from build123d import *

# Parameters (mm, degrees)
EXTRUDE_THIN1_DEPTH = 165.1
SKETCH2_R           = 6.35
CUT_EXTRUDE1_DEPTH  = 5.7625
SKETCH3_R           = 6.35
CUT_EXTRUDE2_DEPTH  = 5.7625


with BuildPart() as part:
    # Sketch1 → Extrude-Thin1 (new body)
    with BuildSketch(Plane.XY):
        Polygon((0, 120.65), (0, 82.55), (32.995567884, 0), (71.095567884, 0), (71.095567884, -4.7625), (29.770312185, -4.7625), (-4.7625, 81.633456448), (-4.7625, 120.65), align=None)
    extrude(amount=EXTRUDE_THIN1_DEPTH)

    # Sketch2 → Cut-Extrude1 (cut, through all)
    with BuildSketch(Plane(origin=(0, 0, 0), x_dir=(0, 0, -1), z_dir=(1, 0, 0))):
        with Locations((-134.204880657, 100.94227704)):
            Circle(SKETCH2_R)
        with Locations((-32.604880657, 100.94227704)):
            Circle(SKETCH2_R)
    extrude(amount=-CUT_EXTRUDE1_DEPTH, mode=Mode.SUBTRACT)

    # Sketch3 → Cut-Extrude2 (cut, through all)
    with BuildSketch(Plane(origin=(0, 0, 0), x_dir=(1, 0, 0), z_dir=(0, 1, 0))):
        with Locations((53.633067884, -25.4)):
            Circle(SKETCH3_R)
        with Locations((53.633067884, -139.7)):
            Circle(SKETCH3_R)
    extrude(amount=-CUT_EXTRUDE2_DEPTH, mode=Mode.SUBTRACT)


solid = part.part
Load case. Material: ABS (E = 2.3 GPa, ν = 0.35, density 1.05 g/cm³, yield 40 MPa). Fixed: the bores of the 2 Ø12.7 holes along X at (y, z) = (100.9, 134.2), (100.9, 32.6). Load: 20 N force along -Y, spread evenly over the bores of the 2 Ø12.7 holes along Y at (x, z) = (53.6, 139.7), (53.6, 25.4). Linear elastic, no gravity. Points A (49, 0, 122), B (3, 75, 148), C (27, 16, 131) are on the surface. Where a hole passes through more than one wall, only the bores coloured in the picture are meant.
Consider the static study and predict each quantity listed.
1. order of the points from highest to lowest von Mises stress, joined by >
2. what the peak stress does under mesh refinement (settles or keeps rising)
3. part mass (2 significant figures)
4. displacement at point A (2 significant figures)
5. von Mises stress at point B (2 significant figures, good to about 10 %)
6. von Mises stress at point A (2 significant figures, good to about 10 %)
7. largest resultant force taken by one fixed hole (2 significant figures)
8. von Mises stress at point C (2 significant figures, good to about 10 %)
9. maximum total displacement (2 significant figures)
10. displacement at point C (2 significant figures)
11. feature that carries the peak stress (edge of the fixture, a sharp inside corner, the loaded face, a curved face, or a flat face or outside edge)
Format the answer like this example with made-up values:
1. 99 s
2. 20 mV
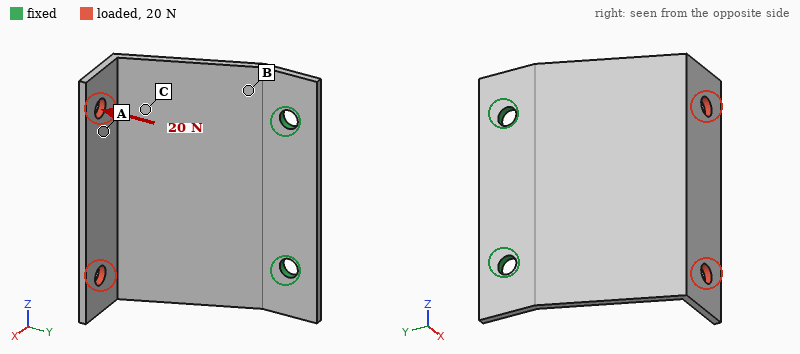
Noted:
1. B > C > A
2. keeps rising
3. 140 g
4. 1.8 mm
5. 1.7 MPa
6. 0.36 MPa
7. 11 N
8. 0.93 MPa
9. 2.3 mm
10. 1.2 mm
11. edge of the fixture
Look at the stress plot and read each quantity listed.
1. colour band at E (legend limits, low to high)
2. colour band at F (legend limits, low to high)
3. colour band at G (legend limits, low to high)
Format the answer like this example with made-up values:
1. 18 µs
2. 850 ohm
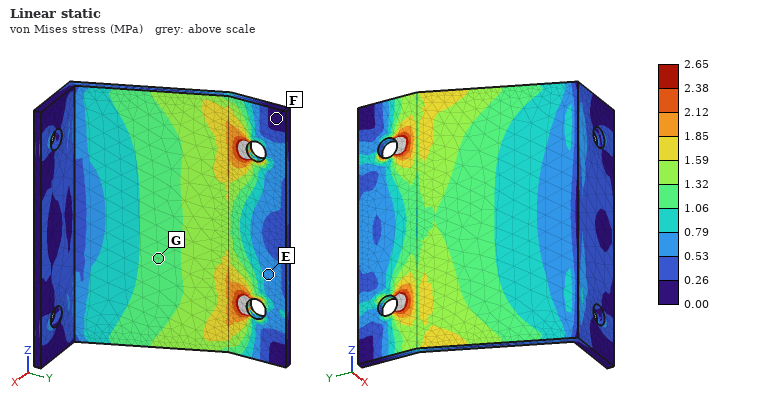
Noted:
1. 0.53 to 0.79 MPa
2. 0.00 to 0.26 MPa
3. 1.06 to 1.32 MPa
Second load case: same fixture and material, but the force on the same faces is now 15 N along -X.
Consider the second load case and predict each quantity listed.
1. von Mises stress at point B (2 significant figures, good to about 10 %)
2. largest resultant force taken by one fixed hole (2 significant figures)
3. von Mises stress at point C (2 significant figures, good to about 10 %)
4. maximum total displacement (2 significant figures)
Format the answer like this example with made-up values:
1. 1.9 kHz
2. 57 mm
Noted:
1. 1.8 MPa
2. 8.1 N
3. 0.41 MPa
4. 2.3 mm
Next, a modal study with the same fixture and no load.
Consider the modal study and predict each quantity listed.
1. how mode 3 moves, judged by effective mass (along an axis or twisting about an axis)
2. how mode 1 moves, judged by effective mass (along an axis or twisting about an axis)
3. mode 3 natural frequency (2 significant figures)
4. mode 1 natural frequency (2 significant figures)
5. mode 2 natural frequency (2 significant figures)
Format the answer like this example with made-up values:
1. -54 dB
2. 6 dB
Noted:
1. along X
2. along X
3. 310 Hz
4. 58 Hz
5. 120 Hz
